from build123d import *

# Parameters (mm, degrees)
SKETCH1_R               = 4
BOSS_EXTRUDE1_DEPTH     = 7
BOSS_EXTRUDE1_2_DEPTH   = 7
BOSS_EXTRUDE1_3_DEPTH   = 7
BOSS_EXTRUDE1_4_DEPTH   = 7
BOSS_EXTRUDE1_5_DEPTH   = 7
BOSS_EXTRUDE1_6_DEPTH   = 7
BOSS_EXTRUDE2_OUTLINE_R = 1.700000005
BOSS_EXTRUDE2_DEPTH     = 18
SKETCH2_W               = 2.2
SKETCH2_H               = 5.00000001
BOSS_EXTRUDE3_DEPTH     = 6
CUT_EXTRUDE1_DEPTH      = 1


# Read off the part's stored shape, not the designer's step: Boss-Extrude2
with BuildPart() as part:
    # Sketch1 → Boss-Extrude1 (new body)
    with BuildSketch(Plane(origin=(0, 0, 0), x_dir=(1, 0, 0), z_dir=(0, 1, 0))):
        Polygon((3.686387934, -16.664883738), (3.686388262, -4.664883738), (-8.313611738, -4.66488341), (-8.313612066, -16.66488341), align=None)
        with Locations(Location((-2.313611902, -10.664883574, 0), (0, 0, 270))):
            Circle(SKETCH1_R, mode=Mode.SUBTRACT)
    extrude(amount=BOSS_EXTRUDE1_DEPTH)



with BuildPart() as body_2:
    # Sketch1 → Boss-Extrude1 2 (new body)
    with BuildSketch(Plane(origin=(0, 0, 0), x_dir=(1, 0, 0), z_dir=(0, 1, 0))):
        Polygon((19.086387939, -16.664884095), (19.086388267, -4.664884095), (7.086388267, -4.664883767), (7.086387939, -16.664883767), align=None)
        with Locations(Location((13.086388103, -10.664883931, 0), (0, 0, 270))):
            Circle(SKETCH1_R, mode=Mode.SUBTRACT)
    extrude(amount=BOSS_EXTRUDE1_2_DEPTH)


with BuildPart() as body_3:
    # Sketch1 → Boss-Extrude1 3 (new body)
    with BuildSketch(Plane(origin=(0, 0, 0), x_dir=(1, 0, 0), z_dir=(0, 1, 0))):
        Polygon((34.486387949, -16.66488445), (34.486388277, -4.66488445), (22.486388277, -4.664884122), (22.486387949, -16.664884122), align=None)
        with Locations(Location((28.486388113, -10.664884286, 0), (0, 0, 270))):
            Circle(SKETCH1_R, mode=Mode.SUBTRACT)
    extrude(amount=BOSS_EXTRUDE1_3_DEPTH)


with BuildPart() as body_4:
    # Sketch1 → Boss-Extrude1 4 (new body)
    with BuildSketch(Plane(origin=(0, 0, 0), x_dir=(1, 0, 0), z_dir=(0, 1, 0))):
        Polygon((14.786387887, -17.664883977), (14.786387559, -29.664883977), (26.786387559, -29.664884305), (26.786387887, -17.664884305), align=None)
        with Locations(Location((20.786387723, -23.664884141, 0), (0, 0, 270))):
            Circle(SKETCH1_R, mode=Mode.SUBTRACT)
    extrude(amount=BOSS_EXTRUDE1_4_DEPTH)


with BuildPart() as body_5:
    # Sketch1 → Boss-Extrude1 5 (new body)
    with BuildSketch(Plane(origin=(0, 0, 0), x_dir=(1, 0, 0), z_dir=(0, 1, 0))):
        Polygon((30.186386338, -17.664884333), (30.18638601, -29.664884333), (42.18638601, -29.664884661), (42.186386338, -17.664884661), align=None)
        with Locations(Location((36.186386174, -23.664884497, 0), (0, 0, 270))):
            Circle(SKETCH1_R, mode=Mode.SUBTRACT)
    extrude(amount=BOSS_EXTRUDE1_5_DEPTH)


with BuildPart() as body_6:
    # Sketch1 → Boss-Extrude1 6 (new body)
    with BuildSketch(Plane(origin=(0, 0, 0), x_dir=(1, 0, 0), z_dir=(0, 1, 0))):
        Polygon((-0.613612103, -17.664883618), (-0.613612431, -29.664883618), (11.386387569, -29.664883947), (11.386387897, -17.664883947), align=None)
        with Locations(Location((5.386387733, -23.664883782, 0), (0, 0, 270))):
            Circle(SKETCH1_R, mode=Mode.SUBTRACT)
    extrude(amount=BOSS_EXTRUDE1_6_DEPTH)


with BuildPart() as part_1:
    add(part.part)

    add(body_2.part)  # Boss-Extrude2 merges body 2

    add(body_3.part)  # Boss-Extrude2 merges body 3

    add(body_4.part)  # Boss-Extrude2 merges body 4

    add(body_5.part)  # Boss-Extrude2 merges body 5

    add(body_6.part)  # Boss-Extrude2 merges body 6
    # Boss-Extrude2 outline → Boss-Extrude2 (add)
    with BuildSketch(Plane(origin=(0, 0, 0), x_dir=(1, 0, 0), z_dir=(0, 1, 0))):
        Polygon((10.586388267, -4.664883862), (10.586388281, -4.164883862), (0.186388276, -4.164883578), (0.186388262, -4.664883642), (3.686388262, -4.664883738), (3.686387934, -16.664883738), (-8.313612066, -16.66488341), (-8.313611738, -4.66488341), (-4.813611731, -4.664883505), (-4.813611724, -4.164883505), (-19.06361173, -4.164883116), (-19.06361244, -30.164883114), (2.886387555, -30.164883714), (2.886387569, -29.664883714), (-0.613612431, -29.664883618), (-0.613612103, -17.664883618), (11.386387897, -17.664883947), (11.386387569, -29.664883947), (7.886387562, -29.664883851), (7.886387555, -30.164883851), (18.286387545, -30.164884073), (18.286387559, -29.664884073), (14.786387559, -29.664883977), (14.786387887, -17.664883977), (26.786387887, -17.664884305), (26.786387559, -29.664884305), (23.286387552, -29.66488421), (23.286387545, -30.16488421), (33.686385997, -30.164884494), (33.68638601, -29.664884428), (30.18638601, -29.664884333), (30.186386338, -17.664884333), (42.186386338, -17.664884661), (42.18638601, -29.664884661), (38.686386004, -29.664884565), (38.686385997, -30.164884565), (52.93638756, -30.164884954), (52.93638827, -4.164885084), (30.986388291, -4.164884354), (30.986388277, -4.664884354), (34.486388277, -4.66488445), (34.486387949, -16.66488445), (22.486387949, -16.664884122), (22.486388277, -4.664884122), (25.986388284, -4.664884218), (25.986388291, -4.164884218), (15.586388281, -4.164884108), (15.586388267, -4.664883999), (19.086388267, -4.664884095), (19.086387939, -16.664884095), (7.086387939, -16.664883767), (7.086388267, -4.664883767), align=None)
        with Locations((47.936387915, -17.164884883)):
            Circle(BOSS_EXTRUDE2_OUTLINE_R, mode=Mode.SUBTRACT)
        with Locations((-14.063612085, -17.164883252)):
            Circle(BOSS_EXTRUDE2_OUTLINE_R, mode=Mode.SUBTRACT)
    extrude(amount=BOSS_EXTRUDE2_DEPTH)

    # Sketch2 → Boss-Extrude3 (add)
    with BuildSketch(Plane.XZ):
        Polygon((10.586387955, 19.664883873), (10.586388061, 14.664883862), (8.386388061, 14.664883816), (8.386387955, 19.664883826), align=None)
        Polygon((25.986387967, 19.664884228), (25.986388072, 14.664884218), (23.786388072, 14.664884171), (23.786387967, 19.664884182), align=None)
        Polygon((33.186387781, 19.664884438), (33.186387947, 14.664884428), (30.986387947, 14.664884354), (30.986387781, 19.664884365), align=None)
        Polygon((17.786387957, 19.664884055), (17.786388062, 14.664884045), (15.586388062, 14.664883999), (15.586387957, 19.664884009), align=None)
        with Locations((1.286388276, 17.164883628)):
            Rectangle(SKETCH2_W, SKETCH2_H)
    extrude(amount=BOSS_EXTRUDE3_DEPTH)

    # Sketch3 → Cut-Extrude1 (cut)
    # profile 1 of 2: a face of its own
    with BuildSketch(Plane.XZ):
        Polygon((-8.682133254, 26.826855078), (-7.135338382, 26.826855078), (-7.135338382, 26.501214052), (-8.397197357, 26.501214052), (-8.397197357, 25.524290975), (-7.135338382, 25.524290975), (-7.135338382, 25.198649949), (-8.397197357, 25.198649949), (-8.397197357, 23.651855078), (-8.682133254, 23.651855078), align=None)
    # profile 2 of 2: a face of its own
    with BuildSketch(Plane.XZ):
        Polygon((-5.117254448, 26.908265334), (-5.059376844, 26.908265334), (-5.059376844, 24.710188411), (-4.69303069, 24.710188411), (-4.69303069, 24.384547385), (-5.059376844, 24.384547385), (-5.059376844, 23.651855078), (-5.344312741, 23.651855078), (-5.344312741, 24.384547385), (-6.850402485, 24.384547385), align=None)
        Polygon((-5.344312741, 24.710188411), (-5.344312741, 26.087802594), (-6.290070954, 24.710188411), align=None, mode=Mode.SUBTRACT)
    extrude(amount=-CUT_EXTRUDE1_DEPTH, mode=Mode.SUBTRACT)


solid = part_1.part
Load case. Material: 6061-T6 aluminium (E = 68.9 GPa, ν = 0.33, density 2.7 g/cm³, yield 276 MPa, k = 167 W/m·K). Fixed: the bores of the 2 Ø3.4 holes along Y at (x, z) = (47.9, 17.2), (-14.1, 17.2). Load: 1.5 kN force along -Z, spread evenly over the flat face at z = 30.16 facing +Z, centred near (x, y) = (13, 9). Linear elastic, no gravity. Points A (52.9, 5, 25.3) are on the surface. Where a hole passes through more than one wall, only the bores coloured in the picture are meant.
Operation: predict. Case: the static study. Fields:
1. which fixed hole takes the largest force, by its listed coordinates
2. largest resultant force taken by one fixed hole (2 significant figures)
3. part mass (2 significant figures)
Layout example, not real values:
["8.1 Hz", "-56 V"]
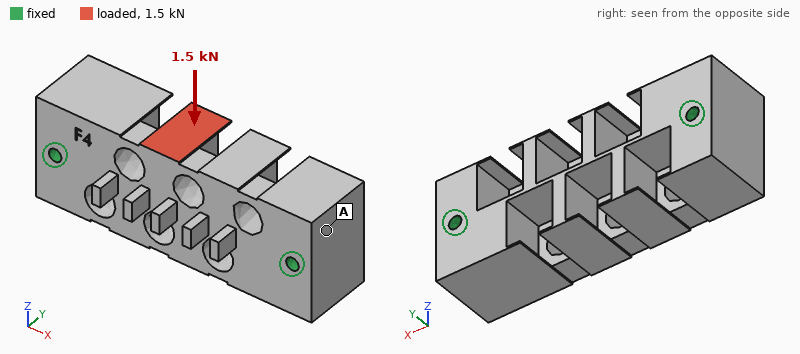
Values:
["(-14.1, 17.2)", "860 N", "59 g"]
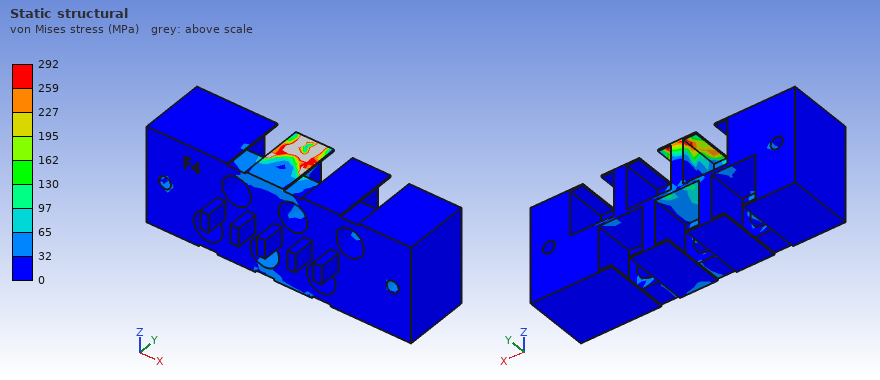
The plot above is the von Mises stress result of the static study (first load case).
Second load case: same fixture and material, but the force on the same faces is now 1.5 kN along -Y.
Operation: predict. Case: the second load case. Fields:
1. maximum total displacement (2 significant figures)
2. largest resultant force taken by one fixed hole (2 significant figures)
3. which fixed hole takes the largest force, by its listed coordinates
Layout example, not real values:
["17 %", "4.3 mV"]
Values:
["96 µm", "1000 N", "(-14.1, 17.2)"]
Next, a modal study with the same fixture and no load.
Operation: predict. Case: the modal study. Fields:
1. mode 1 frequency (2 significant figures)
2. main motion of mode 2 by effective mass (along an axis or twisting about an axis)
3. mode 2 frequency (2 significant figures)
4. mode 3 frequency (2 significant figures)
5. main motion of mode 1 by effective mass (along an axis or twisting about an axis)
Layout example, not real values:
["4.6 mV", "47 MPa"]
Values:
["10 kHz", "along Y", "11 kHz", "13 kHz", "along Z"]
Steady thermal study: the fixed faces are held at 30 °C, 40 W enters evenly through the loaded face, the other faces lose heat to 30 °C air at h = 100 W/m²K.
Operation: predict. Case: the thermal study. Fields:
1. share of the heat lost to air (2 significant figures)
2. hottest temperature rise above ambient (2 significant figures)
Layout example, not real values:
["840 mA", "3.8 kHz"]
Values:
["22 %", "67 K"]
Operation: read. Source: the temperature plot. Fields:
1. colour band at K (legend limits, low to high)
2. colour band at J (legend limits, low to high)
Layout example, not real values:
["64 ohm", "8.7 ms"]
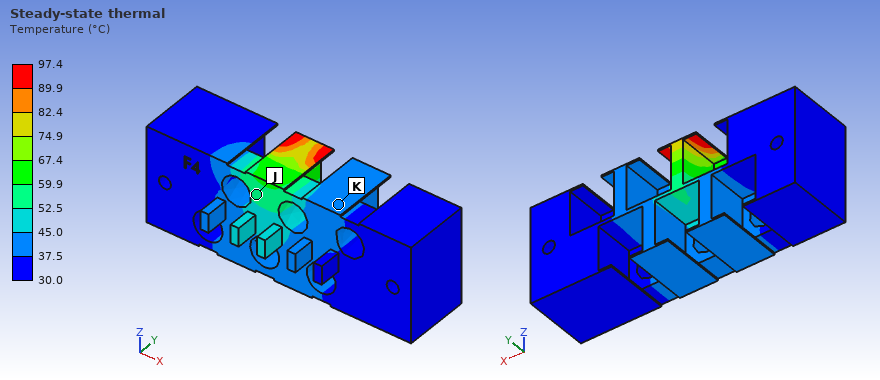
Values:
["37.5 to 45.0 °C", "52.5 to 59.9 °C"]
